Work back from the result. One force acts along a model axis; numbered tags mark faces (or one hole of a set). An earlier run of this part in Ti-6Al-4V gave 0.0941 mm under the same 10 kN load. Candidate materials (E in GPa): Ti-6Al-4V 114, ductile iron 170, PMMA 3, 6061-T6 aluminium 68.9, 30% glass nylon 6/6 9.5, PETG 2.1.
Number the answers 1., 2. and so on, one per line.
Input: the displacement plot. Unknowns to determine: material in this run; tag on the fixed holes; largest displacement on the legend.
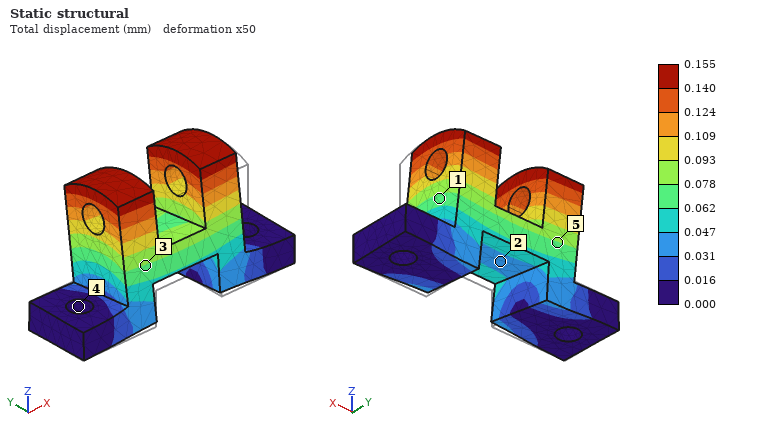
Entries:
1. 6061-T6 aluminium
2. 4
3. 0.155 mm
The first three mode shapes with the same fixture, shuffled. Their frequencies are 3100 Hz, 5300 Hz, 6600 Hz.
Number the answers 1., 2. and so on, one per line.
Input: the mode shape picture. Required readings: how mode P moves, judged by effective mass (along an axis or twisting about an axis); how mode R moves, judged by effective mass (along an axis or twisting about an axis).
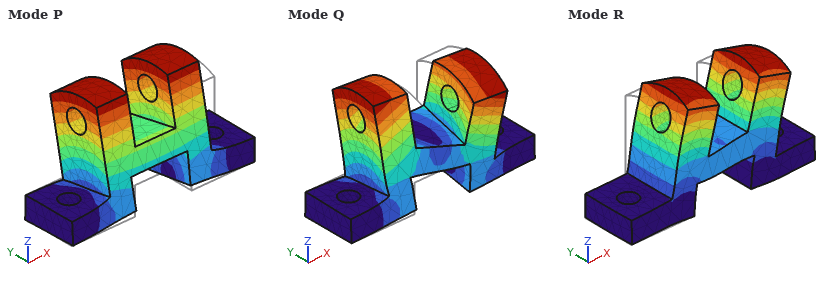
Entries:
1. along Y
2. along X
